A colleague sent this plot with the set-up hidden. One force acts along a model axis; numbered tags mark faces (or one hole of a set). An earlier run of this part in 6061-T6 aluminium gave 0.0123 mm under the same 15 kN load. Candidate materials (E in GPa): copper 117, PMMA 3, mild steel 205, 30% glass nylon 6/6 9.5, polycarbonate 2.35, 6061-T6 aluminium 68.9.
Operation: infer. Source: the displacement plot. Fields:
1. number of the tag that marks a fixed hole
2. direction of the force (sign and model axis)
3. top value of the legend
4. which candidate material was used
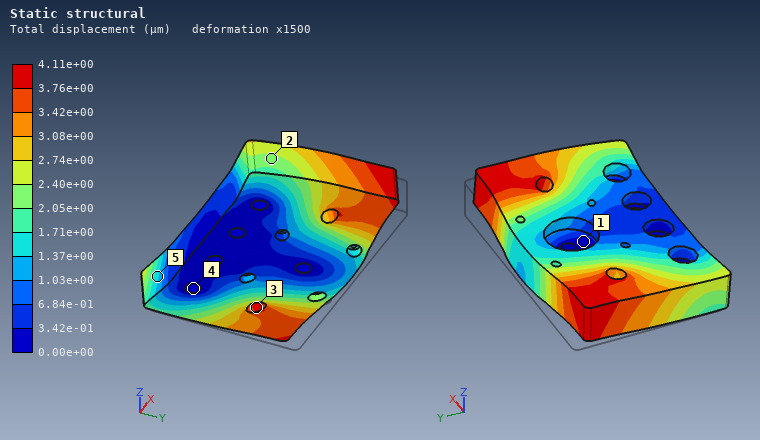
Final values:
4
-Y
4.11e+00 µm
mild steel
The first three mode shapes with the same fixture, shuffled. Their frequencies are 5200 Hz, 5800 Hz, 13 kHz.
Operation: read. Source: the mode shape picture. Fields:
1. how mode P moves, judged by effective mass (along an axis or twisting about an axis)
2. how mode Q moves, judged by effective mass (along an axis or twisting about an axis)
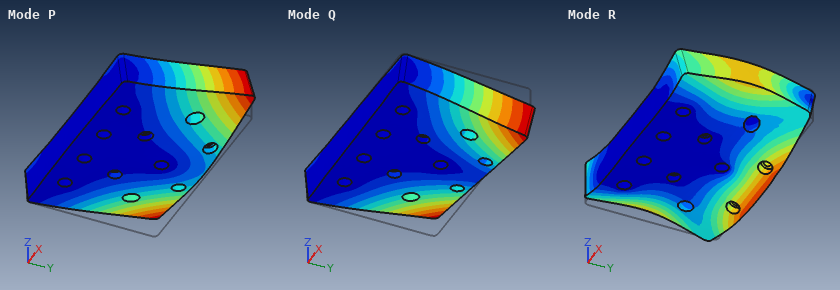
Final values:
along Z
twisting about Y
